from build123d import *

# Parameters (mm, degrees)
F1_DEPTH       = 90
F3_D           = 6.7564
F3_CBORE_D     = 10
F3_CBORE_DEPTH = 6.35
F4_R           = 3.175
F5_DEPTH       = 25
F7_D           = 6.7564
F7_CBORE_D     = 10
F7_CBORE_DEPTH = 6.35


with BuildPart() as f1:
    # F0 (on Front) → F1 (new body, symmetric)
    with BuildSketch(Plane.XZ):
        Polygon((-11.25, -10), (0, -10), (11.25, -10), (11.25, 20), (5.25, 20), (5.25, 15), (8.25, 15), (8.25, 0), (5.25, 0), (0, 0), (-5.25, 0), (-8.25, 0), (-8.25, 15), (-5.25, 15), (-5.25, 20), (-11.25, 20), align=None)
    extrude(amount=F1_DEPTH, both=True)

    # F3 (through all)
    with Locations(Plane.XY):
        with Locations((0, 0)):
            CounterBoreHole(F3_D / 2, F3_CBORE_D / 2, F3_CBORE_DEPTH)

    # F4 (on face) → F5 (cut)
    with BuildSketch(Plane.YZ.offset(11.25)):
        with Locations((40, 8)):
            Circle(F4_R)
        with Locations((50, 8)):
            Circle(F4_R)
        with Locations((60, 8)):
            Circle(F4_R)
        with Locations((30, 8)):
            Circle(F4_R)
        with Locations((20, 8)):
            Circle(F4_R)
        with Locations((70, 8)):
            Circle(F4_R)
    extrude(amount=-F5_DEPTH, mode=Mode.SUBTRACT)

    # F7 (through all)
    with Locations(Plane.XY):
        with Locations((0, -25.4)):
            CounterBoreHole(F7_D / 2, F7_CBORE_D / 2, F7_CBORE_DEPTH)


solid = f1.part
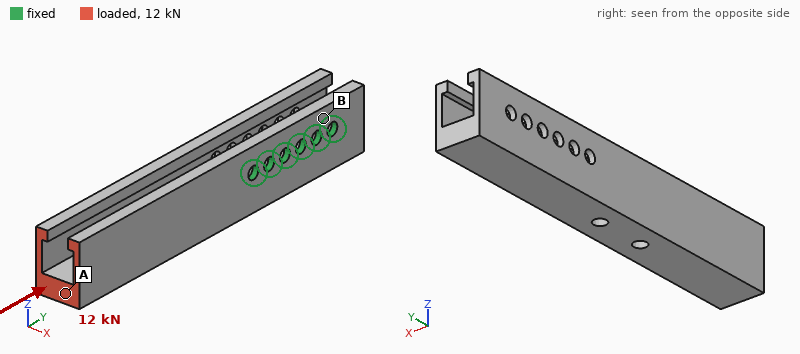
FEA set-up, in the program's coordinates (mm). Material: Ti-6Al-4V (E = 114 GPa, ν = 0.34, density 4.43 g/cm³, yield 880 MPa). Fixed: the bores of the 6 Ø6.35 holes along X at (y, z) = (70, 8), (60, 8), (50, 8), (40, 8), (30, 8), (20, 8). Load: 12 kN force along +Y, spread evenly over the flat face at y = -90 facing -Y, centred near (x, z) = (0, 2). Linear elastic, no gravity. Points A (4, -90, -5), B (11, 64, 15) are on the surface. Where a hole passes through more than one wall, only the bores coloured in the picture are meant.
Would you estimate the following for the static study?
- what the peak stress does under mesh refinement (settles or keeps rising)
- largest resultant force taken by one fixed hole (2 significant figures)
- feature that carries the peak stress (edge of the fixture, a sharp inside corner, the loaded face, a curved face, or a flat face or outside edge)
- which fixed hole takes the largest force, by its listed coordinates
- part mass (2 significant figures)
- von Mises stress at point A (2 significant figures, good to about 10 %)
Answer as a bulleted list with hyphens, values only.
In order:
- keeps rising
- 4.8 kN
- edge of the fixture
- (20, 8)
- 290 g
- 32 MPa
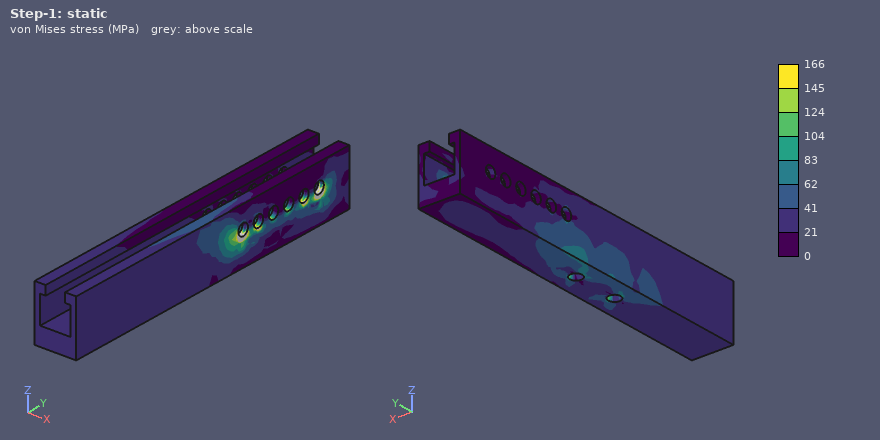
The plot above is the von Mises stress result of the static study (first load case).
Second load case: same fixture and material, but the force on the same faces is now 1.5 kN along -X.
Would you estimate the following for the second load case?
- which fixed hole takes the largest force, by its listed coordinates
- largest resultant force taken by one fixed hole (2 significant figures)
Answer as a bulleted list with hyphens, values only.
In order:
- (20, 8)
- 5.3 kN
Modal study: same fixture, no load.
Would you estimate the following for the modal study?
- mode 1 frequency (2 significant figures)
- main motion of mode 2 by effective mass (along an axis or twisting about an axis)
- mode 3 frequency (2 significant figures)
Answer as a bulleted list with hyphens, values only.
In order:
- 820 Hz
- along Z
- 1600 Hz
